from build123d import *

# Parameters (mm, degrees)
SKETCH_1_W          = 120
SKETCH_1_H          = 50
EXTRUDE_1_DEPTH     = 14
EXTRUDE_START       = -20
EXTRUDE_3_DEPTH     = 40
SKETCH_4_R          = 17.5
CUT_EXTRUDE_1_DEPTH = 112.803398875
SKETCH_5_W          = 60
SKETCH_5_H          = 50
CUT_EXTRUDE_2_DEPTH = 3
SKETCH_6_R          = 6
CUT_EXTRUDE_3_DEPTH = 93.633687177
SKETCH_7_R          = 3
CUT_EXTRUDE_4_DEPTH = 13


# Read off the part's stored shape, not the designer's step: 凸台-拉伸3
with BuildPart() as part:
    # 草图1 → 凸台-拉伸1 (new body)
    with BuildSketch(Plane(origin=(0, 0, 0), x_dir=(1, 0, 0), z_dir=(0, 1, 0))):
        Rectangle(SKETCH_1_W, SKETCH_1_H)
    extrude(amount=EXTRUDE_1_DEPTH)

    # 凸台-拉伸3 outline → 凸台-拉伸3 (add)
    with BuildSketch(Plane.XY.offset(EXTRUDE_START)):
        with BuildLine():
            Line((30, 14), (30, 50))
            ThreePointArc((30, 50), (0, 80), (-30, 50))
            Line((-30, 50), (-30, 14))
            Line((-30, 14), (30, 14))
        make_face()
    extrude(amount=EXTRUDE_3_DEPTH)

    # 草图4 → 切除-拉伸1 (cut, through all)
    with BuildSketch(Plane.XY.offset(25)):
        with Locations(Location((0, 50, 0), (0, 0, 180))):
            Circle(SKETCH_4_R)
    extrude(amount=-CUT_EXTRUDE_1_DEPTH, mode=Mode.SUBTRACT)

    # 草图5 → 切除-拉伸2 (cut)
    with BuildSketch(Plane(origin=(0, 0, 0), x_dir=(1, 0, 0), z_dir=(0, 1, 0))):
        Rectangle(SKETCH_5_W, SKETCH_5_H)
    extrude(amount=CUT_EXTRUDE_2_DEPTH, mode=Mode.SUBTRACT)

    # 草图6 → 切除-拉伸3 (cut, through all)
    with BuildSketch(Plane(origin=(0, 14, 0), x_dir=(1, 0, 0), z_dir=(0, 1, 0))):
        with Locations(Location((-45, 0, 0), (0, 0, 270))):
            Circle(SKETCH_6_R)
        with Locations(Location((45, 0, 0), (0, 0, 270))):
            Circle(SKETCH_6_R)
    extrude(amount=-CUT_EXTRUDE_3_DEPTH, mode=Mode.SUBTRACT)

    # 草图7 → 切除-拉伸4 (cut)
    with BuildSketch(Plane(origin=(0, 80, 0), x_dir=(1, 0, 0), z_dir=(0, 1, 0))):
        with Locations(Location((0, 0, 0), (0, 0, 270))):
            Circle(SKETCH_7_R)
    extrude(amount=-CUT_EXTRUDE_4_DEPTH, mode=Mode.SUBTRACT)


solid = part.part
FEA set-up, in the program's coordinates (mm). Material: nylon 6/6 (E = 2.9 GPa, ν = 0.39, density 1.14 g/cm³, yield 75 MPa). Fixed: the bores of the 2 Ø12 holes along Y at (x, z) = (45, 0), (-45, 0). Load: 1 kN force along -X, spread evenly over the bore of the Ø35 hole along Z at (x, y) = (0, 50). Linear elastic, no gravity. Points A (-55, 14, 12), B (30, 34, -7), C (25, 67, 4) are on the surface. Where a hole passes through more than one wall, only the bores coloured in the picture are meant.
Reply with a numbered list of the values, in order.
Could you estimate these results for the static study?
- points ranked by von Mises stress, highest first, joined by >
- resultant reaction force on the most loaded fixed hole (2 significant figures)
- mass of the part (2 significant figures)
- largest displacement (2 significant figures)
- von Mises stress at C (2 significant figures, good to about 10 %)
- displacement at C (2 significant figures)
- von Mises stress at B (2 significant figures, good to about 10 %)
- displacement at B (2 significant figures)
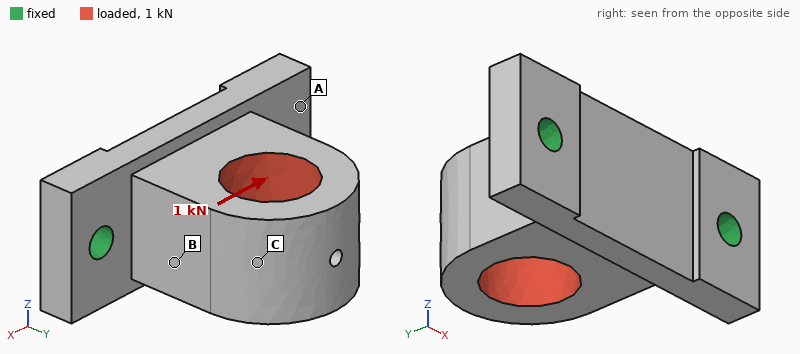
1. B > C > A
2. 780 N
3. 200 g
4. 0.16 mm
5. 1.1 MPa
6. 0.14 mm
7. 2.0 MPa
8. 0.062 mm
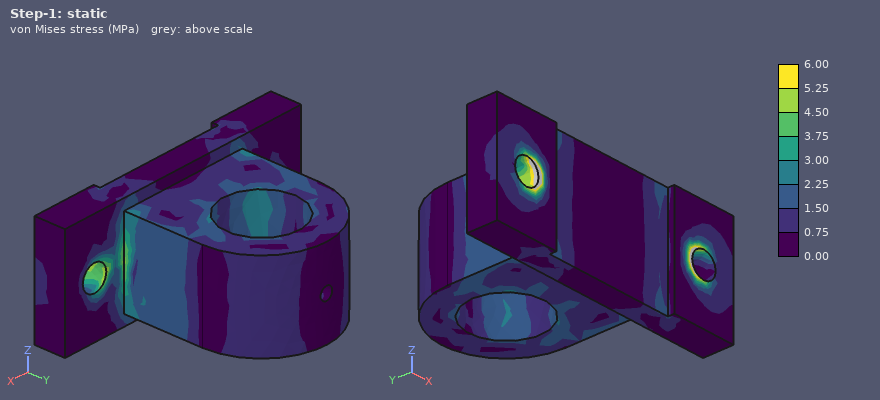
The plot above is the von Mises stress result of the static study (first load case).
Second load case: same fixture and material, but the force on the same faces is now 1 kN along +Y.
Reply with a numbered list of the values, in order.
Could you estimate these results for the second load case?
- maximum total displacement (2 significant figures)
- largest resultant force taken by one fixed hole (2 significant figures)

1. 49 µm
2. 560 N
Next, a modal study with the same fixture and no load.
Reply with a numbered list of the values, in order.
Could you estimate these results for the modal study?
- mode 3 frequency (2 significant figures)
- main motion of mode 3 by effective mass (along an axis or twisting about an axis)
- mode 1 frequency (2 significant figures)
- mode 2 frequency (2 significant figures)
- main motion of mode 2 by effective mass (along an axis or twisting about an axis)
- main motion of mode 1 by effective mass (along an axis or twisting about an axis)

1. 2100 Hz
2. along Y
3. 700 Hz
4. 1500 Hz
5. along X
6. along Z
